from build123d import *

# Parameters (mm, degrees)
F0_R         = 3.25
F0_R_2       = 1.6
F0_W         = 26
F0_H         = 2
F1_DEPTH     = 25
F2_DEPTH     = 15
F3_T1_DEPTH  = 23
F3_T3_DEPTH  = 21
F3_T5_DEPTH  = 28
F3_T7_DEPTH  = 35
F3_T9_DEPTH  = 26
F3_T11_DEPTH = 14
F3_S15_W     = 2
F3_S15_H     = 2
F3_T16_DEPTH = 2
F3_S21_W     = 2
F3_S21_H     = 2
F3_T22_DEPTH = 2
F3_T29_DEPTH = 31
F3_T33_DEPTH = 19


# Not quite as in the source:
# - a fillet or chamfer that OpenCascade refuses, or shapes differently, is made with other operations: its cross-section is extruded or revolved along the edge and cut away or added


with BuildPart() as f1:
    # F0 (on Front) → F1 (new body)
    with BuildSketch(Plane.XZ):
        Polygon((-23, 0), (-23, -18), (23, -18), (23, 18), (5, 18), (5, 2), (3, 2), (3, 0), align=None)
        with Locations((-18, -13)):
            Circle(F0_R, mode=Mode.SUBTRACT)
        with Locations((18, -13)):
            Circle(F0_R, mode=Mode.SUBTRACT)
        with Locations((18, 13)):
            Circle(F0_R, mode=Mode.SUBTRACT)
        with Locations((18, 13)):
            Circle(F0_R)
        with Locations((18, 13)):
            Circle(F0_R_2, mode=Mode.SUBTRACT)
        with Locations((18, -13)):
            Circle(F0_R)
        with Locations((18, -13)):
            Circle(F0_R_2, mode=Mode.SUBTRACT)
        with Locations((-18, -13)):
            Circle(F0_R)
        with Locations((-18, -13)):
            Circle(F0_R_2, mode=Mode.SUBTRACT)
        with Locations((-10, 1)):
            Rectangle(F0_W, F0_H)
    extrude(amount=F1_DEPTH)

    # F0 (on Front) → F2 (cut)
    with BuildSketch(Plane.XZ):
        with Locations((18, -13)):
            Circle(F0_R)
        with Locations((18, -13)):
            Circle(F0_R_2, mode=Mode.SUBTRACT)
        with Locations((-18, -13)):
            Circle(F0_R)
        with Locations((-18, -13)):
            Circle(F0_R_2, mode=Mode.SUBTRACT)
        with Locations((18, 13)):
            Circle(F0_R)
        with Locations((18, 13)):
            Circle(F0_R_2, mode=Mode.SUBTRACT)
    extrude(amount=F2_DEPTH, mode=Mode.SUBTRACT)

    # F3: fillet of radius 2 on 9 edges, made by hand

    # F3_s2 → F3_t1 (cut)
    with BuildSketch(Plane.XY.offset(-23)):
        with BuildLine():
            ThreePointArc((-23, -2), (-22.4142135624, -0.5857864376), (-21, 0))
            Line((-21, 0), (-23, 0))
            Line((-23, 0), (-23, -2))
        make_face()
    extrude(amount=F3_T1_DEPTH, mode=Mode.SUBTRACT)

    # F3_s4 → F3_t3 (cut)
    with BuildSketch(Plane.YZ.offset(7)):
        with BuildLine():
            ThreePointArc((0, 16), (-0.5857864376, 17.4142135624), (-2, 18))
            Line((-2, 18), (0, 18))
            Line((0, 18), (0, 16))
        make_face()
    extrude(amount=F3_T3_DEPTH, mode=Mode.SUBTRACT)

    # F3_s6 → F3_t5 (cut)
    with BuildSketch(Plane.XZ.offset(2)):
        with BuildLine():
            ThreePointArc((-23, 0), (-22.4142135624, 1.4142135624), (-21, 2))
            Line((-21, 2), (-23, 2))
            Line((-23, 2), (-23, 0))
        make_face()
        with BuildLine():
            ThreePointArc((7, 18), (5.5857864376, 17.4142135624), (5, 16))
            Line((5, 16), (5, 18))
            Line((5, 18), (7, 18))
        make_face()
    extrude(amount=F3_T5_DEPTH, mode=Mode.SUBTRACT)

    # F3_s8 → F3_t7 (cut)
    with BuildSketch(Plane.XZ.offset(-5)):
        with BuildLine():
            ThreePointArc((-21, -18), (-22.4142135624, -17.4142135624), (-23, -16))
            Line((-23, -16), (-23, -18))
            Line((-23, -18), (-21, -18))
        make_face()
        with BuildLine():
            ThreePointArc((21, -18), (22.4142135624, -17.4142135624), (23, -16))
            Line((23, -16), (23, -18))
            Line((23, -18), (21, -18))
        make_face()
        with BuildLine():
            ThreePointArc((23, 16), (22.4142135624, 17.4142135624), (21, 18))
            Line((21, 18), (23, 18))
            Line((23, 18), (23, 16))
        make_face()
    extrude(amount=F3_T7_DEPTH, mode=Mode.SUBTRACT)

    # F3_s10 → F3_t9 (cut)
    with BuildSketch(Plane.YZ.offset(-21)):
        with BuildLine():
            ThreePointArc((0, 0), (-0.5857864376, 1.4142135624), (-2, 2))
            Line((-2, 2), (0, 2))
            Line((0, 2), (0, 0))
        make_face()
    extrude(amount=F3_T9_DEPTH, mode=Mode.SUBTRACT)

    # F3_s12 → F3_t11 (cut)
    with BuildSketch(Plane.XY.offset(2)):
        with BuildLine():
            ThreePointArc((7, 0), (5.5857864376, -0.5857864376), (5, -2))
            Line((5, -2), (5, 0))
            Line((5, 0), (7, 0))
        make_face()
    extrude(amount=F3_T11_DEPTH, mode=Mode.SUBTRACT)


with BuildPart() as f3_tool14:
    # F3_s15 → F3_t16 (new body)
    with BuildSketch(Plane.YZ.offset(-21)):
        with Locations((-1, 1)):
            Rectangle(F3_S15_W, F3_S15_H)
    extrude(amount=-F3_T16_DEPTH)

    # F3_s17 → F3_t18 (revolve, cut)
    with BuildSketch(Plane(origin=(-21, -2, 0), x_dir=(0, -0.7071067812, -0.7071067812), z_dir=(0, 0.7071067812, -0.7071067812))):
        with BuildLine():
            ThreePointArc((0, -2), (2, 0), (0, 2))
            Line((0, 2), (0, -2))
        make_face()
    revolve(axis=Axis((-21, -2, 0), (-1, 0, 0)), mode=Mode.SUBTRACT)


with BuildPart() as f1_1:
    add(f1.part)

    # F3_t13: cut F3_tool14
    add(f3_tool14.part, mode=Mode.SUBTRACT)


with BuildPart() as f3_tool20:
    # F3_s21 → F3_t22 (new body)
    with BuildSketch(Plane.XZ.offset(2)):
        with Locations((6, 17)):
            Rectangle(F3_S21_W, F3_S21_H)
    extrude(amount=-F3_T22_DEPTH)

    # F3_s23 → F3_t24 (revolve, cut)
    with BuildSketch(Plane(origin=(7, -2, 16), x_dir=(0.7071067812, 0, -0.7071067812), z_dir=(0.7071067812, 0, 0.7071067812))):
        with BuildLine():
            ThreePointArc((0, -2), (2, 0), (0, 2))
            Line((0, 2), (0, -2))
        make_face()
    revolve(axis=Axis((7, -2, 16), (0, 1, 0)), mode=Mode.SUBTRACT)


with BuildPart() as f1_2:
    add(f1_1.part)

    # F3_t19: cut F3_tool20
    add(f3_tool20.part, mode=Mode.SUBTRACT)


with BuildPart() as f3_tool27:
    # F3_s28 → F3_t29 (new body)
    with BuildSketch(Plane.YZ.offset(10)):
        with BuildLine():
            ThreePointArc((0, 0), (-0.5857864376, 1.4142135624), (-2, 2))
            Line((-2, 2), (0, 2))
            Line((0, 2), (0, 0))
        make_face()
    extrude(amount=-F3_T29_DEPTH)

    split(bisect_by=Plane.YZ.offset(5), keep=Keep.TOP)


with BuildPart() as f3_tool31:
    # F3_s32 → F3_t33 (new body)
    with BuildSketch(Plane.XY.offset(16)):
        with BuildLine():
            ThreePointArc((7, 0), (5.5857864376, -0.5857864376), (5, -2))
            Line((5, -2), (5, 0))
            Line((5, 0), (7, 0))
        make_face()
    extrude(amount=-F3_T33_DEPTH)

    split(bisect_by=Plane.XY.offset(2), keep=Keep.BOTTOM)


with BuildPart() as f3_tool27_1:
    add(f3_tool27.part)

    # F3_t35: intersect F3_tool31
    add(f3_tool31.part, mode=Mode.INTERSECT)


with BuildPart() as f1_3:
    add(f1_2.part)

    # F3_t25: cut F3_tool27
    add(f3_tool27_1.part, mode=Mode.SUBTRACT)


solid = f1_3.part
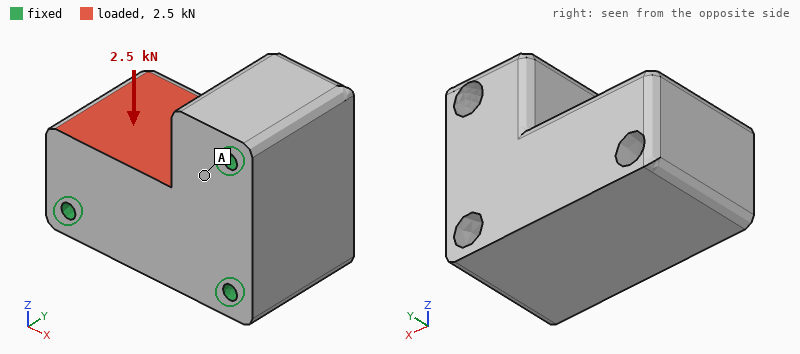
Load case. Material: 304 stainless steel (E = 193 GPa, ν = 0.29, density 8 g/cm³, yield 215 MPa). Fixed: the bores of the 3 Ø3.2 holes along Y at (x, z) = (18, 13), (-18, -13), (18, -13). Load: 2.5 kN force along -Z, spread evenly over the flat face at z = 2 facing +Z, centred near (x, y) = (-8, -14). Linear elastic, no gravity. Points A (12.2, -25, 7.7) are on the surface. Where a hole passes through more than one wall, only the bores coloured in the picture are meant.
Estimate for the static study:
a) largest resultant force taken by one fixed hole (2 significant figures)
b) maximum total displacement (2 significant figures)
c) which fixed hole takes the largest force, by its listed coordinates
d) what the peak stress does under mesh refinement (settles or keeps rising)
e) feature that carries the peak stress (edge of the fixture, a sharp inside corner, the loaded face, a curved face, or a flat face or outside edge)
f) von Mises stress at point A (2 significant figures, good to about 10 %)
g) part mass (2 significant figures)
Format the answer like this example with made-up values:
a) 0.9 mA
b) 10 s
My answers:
a) 1.4 kN
b) 2.4 µm
c) (-18, -13)
d) keeps rising
e) edge of the fixture
f) 4.4 MPa
g) 230 g
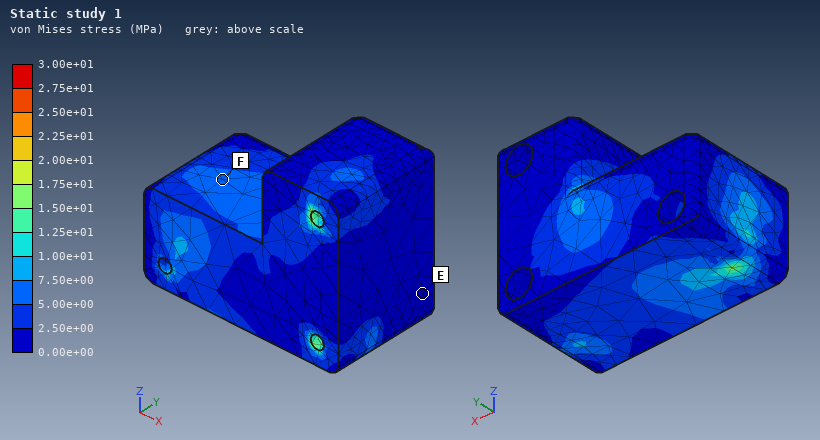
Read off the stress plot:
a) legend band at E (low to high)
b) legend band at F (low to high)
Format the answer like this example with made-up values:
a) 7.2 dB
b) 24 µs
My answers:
a) 0.00e+00 to 2.50e+00 MPa
b) 5.00e+00 to 7.50e+00 MPa
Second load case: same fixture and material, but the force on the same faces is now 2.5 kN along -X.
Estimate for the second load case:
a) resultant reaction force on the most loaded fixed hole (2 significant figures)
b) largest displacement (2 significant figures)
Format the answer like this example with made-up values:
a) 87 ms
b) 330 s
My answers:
a) 1.4 kN
b) 2.0 µm
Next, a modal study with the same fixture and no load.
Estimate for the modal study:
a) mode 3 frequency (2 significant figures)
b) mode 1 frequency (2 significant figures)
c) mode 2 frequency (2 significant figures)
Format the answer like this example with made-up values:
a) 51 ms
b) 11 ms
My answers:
a) 22 kHz
b) 15 kHz
c) 21 kHz
